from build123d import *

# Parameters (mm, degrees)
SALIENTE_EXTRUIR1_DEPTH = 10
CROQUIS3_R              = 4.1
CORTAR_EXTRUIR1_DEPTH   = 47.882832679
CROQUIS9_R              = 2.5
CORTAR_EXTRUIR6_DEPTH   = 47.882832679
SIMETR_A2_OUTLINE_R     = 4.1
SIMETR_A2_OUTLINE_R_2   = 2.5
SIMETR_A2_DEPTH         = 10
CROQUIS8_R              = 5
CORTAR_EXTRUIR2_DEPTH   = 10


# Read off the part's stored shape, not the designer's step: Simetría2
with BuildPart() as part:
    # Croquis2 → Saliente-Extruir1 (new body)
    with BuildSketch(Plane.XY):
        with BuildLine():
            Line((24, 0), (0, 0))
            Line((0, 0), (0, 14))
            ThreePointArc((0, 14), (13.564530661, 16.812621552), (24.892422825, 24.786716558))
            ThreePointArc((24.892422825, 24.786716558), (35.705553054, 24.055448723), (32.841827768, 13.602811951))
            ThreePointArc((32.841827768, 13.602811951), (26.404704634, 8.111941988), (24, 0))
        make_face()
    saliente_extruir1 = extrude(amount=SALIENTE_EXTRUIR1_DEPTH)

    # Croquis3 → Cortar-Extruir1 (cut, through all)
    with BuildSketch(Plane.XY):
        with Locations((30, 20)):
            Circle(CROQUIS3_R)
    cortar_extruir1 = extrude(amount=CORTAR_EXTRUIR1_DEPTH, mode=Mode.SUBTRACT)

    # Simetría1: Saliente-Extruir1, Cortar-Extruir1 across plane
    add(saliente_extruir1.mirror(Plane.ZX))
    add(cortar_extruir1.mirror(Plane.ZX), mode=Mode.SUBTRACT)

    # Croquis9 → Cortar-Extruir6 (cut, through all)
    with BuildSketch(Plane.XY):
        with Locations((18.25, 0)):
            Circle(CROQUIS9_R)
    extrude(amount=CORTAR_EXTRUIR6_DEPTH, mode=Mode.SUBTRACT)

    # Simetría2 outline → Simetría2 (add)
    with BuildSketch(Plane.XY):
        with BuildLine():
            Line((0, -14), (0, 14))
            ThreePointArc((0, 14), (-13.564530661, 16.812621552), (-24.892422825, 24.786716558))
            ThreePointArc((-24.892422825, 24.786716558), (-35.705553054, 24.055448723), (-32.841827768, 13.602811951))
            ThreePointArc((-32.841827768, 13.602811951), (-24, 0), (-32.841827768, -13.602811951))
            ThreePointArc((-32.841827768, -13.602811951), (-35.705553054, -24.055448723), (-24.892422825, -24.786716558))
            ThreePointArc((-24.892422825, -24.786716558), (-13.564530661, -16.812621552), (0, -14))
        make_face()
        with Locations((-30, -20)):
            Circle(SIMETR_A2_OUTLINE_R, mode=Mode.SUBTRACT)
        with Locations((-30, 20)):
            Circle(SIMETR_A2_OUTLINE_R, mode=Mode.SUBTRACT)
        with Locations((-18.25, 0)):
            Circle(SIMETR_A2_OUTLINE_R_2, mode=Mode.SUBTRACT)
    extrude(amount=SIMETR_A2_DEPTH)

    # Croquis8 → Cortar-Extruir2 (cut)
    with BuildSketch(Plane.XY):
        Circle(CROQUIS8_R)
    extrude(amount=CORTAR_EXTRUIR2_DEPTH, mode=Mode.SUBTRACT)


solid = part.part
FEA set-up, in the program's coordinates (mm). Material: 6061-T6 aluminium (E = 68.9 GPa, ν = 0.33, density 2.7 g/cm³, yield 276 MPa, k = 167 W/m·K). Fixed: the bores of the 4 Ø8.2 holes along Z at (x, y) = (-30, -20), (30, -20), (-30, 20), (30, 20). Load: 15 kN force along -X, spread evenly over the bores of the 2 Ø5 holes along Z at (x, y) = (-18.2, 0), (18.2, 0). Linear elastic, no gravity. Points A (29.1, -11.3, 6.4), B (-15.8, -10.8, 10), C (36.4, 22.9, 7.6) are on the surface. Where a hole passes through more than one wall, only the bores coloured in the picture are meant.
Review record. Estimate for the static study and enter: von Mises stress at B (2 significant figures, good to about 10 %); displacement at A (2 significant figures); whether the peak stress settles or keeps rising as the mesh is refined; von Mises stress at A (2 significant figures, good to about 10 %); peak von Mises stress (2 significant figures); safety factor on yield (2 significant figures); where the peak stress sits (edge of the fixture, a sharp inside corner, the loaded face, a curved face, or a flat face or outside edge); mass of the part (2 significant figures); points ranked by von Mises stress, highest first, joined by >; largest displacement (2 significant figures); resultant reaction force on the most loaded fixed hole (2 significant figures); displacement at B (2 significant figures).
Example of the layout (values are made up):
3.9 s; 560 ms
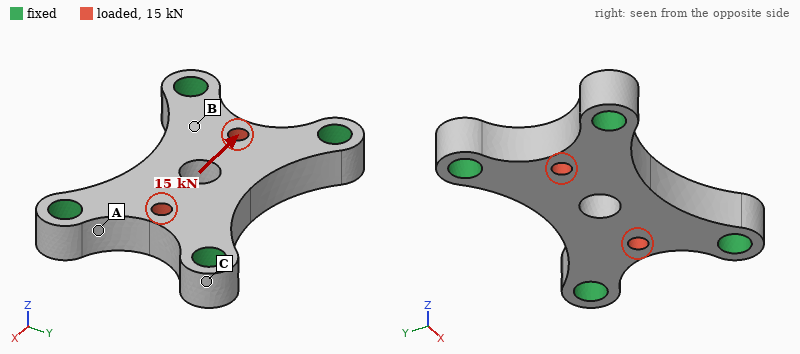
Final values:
27 MPa; 4.8 µm; settles; 57 MPa; 110 MPa; 2.5; the loaded face; 55 g; A > B > C; 22 µm; 4.5 kN; 8.8 µm
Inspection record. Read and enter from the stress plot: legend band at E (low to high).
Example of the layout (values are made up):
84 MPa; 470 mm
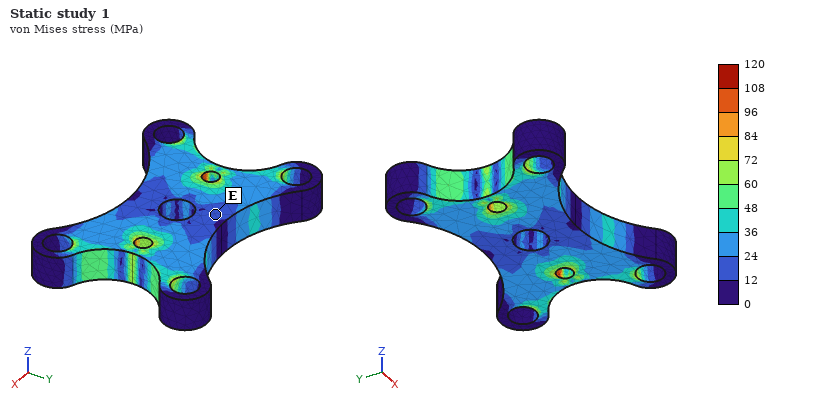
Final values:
12 to 24 MPa
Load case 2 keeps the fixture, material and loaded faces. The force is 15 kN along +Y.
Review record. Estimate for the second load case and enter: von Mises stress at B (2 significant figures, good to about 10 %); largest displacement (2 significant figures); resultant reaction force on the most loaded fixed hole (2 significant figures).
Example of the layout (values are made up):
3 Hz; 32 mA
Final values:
17 MPa; 15 µm; 4.2 kN
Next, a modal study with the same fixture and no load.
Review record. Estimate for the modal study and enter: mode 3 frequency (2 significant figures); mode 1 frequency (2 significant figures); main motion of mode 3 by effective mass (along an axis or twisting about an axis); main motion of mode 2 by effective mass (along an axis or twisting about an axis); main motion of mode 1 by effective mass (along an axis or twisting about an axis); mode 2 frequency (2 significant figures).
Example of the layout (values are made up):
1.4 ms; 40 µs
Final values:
25 kHz; 12 kHz; twisting about Y; twisting about X; along Z; 22 kHz
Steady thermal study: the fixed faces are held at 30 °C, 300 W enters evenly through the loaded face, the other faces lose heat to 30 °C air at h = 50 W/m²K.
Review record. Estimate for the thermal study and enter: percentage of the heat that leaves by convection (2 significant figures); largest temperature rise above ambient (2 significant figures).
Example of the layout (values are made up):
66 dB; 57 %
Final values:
3.3 %; 65 K
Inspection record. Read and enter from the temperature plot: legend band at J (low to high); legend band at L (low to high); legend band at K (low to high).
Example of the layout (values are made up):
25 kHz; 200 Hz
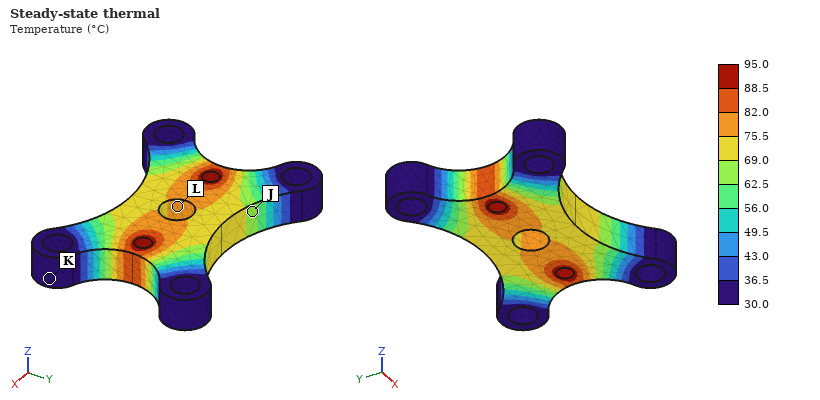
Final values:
62.5 to 69.0 °C; 75.5 to 82.0 °C; 30.0 to 36.5 °C
